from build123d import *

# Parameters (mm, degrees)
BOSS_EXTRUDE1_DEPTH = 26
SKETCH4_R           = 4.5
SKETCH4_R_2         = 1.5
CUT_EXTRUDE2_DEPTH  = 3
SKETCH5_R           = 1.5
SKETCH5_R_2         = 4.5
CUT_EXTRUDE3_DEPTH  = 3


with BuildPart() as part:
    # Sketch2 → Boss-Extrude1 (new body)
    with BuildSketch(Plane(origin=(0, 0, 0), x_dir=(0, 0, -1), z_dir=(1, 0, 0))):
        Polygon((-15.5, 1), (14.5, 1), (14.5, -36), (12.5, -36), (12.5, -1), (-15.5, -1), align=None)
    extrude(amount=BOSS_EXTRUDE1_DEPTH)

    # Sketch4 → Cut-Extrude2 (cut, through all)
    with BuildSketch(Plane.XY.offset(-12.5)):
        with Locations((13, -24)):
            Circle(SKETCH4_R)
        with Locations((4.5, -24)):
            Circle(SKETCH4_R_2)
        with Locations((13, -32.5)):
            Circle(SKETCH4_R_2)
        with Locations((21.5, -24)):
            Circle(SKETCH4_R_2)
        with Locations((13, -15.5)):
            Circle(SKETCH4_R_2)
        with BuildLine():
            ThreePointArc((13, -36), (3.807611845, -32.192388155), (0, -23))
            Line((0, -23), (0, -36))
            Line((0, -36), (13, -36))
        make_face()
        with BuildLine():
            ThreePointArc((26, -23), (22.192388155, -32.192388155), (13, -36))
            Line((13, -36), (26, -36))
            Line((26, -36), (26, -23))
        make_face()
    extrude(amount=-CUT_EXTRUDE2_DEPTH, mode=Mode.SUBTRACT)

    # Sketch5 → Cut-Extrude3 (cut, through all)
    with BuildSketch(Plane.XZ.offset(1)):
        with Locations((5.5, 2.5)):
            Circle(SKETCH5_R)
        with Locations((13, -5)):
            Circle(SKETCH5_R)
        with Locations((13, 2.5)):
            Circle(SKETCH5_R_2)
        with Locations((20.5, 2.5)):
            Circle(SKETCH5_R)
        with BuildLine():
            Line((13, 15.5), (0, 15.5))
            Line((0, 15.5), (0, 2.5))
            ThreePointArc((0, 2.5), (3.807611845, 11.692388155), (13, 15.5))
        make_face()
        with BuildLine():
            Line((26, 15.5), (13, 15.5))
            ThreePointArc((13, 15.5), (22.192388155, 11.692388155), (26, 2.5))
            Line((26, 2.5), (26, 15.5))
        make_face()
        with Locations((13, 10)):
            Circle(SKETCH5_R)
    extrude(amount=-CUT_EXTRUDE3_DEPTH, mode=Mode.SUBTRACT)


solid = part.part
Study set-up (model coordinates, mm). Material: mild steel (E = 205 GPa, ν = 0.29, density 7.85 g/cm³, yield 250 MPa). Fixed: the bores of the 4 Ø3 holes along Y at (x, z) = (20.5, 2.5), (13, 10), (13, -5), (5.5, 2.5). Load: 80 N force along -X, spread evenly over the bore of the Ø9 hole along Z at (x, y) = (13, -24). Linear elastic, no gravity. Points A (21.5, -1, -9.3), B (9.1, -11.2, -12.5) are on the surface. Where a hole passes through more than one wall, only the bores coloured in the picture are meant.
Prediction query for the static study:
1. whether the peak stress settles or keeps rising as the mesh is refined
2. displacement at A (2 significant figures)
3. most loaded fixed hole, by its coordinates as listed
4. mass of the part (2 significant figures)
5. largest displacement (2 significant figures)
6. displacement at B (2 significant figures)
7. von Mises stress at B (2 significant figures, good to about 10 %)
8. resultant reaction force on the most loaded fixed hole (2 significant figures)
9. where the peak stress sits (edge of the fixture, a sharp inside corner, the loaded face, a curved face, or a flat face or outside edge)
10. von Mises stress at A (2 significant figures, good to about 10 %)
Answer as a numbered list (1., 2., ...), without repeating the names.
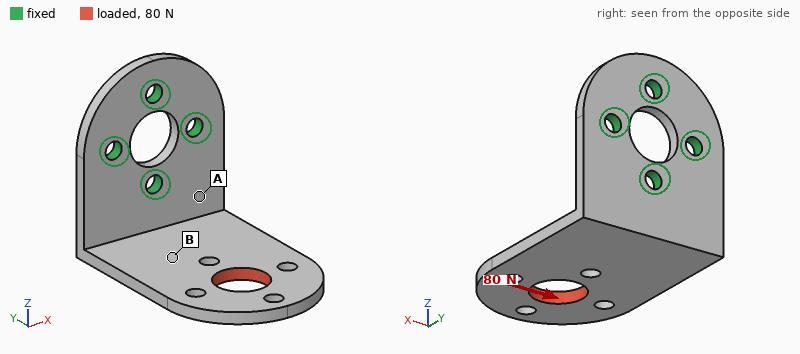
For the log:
1. keeps rising
2. 13 µm
3. (13, -5)
4. 21 g
5. 81 µm
6. 27 µm
7. 11 MPa
8. 79 N
9. edge of the fixture
10. 42 MPa
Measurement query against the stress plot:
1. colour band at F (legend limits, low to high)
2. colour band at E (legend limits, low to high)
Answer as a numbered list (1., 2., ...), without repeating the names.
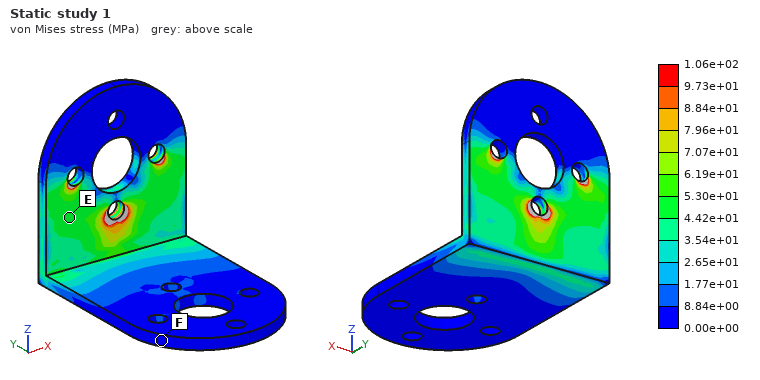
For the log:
1. 0.00e+00 to 8.84e+00 MPa
2. 4.42e+01 to 5.30e+01 MPa
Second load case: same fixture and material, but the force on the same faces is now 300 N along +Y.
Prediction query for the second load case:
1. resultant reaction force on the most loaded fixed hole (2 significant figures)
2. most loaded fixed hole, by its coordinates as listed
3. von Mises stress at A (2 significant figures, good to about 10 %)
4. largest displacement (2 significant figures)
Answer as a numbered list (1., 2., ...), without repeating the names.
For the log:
1. 380 N
2. (13, -5)
3. 57 MPa
4. 0.12 mm
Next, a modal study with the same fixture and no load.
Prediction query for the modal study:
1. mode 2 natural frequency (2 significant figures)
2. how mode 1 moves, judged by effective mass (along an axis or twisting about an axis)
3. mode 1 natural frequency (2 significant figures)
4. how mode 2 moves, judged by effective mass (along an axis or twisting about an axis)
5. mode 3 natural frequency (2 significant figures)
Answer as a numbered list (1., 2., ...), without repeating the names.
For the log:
1. 2100 Hz
2. along Z
3. 1100 Hz
4. along X
5. 4500 Hz
